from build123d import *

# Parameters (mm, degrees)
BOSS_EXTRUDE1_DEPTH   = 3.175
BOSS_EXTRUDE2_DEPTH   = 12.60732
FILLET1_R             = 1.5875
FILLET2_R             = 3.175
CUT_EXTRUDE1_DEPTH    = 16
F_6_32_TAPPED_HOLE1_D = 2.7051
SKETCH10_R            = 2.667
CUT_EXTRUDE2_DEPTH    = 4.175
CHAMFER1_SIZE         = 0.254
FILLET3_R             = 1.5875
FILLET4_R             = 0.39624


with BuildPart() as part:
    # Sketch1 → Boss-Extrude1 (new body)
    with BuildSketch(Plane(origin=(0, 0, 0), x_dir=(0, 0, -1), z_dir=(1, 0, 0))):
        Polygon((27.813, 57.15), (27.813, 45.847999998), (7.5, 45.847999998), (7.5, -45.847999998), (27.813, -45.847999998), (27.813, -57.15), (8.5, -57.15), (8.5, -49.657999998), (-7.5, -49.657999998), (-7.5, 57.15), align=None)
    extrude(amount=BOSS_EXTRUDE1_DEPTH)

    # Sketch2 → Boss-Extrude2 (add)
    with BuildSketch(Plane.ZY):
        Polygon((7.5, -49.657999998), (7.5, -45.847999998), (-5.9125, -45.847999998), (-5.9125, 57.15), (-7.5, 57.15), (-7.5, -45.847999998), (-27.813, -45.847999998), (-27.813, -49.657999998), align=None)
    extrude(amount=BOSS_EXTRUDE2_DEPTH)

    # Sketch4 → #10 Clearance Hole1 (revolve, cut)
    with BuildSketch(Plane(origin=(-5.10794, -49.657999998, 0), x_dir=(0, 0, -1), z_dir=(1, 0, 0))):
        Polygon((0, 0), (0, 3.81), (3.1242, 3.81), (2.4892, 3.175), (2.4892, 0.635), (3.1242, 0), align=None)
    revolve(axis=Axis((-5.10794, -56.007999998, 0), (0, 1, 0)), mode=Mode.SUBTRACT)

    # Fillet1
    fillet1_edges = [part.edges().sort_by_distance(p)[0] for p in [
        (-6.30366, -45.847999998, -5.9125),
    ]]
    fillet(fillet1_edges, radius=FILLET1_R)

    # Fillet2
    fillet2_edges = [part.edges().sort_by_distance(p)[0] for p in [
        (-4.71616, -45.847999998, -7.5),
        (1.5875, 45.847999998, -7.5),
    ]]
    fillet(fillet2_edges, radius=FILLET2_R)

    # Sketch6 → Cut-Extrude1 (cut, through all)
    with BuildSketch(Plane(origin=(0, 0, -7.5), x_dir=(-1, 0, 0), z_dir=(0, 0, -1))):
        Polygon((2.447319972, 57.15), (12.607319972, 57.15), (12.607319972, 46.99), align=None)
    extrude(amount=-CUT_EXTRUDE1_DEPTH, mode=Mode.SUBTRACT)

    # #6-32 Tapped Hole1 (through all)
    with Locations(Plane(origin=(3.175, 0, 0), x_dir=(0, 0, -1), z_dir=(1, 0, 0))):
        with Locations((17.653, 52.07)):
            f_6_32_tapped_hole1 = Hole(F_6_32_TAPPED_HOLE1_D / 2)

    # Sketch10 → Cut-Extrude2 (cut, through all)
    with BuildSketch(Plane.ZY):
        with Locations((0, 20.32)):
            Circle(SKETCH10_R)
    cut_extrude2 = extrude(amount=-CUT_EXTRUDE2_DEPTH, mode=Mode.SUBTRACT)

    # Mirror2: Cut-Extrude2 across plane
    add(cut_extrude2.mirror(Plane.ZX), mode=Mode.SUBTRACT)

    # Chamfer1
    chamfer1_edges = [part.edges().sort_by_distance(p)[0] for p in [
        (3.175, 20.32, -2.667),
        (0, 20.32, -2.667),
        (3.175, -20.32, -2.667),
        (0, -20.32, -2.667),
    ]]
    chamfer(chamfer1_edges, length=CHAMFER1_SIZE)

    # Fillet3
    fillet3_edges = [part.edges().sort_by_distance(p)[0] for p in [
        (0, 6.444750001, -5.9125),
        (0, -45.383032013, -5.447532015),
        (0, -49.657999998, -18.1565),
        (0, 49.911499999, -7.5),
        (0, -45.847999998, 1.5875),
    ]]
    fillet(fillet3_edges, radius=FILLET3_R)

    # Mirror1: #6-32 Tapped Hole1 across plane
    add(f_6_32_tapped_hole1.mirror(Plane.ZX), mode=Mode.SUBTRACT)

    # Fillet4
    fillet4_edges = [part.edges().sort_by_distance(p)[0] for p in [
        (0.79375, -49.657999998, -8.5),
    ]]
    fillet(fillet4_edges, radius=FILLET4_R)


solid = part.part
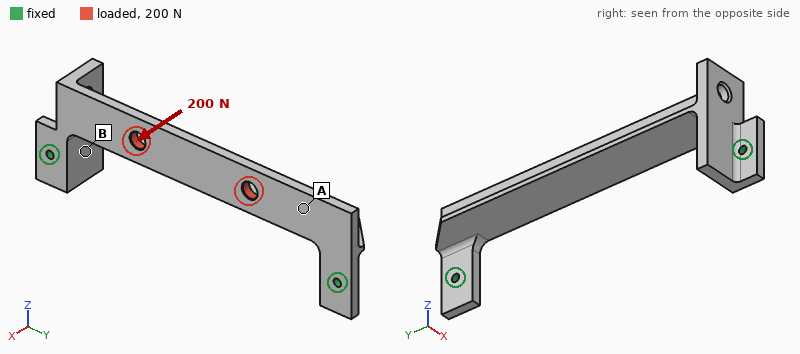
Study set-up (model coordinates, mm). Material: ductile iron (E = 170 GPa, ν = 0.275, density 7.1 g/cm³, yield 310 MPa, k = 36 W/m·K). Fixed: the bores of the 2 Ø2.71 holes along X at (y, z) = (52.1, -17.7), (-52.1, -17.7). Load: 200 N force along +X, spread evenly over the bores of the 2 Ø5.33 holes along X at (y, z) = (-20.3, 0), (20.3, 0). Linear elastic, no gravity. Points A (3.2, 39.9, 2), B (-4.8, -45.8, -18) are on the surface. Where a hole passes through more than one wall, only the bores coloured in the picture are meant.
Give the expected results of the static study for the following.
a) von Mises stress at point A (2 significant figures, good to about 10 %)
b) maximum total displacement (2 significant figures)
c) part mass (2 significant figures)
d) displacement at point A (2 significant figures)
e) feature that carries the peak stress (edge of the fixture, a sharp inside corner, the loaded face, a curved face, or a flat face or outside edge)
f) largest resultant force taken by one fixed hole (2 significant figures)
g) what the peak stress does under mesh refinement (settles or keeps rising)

11 MPa
71 µm
71 g
41 µm
edge of the fixture
130 N
keeps rising
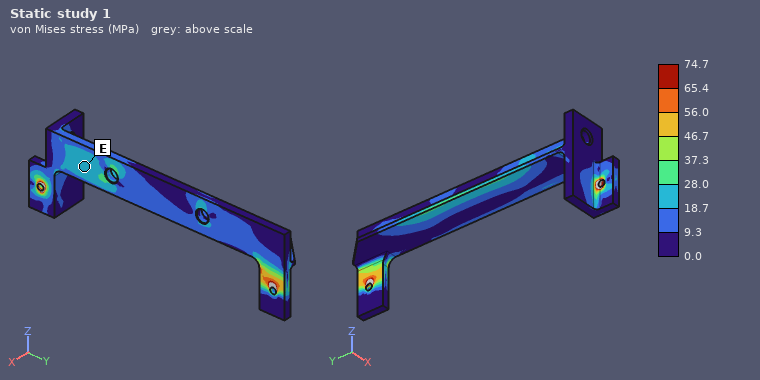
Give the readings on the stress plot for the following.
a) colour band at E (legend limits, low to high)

18.7 to 28.0 MPa
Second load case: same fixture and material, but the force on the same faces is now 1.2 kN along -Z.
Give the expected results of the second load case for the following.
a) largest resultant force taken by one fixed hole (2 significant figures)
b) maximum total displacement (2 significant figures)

910 N
51 µm
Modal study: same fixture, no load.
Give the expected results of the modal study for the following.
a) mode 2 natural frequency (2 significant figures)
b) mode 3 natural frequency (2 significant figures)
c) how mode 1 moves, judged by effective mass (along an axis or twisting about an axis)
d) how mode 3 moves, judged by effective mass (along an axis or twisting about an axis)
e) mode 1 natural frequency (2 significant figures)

3300 Hz
3700 Hz
along X
along Z
1700 Hz
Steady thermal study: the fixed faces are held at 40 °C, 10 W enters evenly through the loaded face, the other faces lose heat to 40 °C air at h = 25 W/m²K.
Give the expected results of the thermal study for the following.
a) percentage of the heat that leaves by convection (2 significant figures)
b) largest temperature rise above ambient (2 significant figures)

60 %
58 K
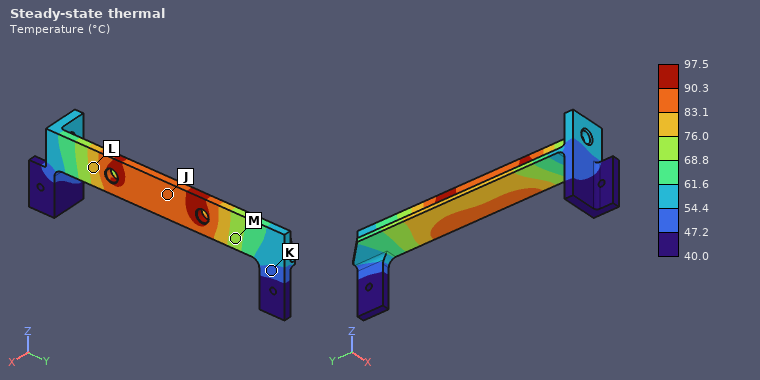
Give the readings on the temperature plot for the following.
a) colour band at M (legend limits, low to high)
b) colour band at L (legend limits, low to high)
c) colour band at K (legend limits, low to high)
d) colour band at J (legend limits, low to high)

68.8 to 76.0 °C
76.0 to 83.1 °C
47.2 to 54.4 °C
83.1 to 90.3 °C
